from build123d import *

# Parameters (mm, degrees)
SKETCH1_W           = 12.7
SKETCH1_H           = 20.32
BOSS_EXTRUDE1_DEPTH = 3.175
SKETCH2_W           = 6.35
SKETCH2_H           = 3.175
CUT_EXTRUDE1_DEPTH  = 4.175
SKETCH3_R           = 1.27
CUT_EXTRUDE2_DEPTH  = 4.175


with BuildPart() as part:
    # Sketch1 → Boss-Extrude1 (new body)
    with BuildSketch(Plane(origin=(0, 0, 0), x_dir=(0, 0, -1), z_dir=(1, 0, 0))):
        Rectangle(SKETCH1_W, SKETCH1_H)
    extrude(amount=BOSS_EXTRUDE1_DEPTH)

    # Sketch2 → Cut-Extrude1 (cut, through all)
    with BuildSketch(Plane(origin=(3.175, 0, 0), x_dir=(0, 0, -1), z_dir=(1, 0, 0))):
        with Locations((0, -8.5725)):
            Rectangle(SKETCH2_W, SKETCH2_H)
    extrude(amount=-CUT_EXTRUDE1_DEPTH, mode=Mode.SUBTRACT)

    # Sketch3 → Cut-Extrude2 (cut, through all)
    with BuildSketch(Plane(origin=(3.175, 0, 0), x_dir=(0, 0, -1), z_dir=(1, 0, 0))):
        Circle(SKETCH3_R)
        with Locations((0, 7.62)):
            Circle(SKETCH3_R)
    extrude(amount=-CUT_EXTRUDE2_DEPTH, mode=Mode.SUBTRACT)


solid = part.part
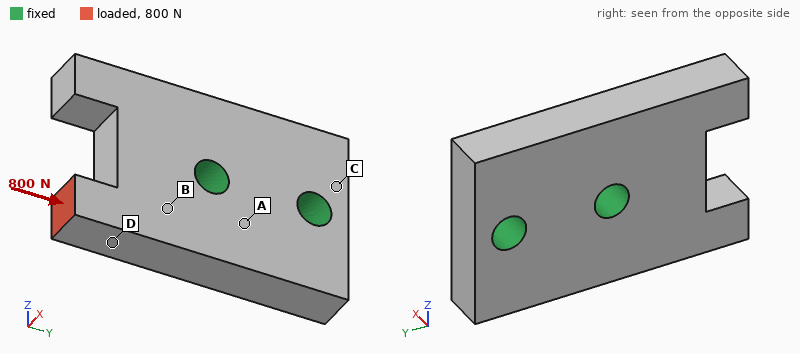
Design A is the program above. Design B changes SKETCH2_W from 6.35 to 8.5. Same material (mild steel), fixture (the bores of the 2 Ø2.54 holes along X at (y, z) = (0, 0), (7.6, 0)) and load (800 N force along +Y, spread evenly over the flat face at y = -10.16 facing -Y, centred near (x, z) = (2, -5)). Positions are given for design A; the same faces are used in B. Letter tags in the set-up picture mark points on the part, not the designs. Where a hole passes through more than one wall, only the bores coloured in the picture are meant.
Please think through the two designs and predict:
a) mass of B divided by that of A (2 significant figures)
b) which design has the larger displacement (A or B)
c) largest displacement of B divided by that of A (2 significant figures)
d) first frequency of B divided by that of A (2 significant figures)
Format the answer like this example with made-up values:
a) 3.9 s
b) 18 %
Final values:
a) 0.97
b) B
c) 1.3
d) 1.1
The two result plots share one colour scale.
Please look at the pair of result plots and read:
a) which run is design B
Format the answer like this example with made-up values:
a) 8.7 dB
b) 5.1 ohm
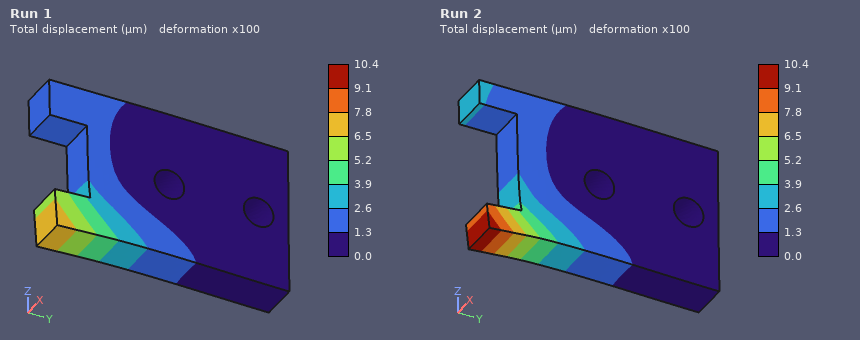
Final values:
a) Run 2
